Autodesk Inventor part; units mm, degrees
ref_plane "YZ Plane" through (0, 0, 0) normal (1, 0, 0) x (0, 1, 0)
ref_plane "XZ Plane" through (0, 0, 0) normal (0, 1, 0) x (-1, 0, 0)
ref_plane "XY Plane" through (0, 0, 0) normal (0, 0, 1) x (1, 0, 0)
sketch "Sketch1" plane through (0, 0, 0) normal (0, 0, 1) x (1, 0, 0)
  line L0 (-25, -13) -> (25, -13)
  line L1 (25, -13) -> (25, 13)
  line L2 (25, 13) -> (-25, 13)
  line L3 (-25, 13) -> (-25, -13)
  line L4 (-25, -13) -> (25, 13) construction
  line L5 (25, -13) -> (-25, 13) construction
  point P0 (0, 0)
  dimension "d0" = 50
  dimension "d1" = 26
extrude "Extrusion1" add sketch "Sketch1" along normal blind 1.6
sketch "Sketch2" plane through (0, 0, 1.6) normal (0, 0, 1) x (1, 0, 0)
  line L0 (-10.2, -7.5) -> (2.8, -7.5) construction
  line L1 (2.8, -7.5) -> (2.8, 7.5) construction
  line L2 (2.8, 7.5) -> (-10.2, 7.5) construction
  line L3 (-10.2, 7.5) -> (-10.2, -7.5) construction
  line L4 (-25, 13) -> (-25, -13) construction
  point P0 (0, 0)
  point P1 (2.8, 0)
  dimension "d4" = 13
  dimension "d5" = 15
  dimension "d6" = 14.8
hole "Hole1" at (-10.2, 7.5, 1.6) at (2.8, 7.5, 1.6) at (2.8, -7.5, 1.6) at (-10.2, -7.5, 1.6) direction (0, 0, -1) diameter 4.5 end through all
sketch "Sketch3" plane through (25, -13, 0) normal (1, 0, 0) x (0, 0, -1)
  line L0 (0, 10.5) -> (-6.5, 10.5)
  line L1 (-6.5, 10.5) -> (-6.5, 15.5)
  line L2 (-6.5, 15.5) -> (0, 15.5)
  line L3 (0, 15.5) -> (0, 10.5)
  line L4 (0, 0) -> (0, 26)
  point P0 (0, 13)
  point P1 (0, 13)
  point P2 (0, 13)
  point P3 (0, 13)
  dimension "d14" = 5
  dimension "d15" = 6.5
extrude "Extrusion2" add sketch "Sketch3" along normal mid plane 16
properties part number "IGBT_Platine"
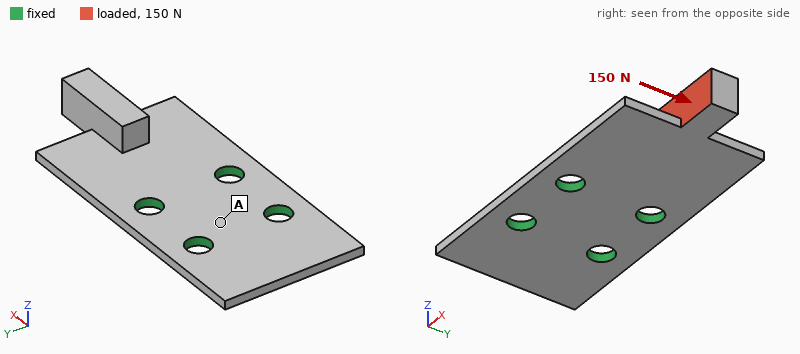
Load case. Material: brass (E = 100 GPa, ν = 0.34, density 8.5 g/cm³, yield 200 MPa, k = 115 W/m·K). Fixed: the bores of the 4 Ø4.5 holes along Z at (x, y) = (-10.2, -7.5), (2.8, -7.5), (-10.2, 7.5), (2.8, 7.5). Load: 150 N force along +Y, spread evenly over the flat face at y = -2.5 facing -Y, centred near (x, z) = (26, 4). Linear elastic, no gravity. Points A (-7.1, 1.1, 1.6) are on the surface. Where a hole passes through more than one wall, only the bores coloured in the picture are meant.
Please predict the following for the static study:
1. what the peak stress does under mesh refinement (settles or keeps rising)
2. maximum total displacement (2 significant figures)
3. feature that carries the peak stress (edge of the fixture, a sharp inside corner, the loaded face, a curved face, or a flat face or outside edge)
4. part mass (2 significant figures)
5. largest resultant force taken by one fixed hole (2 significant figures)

keeps rising
35 µm
edge of the fixture
21 g
190 N
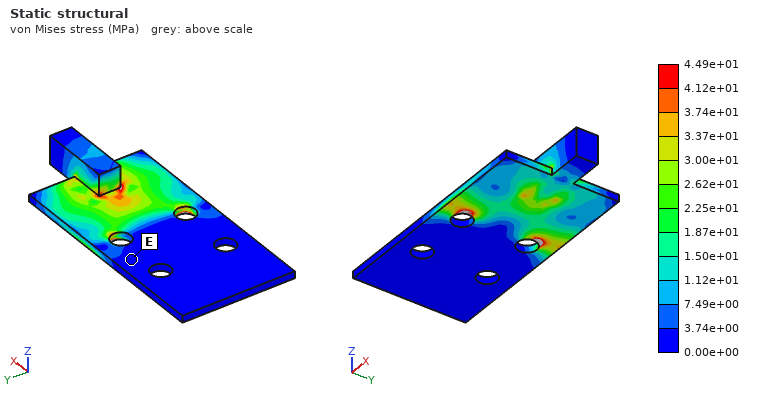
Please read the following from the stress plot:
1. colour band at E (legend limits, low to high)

0.00e+00 to 3.74e+00 MPa
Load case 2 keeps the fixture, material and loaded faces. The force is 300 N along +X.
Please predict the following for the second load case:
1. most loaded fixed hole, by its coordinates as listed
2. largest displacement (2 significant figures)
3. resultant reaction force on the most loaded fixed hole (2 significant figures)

(2.8, -7.5)
0.30 mm
180 N
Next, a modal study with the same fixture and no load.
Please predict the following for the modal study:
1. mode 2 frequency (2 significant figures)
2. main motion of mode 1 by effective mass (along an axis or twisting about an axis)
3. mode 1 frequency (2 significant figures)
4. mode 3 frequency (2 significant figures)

4100 Hz
along Z
1100 Hz
5000 Hz
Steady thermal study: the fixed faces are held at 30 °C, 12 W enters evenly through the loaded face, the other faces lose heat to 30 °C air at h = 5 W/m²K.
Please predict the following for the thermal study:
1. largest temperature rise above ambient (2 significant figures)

66 K
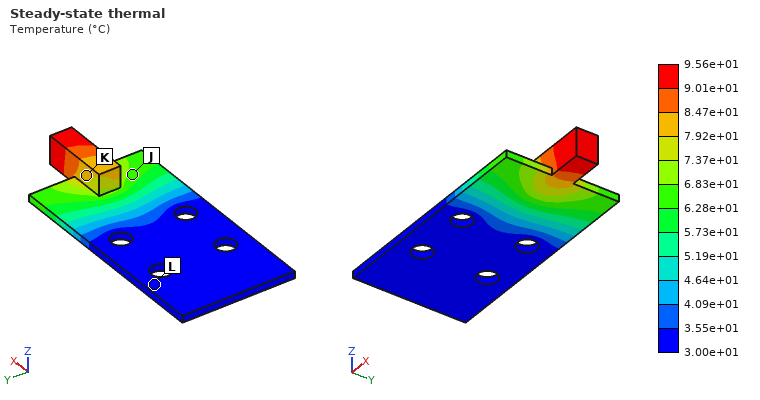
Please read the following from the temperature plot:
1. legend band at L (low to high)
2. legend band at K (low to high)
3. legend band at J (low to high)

3.00e+01 to 3.55e+01 °C
7.92e+01 to 8.47e+01 °C
6.28e+01 to 6.83e+01 °C
